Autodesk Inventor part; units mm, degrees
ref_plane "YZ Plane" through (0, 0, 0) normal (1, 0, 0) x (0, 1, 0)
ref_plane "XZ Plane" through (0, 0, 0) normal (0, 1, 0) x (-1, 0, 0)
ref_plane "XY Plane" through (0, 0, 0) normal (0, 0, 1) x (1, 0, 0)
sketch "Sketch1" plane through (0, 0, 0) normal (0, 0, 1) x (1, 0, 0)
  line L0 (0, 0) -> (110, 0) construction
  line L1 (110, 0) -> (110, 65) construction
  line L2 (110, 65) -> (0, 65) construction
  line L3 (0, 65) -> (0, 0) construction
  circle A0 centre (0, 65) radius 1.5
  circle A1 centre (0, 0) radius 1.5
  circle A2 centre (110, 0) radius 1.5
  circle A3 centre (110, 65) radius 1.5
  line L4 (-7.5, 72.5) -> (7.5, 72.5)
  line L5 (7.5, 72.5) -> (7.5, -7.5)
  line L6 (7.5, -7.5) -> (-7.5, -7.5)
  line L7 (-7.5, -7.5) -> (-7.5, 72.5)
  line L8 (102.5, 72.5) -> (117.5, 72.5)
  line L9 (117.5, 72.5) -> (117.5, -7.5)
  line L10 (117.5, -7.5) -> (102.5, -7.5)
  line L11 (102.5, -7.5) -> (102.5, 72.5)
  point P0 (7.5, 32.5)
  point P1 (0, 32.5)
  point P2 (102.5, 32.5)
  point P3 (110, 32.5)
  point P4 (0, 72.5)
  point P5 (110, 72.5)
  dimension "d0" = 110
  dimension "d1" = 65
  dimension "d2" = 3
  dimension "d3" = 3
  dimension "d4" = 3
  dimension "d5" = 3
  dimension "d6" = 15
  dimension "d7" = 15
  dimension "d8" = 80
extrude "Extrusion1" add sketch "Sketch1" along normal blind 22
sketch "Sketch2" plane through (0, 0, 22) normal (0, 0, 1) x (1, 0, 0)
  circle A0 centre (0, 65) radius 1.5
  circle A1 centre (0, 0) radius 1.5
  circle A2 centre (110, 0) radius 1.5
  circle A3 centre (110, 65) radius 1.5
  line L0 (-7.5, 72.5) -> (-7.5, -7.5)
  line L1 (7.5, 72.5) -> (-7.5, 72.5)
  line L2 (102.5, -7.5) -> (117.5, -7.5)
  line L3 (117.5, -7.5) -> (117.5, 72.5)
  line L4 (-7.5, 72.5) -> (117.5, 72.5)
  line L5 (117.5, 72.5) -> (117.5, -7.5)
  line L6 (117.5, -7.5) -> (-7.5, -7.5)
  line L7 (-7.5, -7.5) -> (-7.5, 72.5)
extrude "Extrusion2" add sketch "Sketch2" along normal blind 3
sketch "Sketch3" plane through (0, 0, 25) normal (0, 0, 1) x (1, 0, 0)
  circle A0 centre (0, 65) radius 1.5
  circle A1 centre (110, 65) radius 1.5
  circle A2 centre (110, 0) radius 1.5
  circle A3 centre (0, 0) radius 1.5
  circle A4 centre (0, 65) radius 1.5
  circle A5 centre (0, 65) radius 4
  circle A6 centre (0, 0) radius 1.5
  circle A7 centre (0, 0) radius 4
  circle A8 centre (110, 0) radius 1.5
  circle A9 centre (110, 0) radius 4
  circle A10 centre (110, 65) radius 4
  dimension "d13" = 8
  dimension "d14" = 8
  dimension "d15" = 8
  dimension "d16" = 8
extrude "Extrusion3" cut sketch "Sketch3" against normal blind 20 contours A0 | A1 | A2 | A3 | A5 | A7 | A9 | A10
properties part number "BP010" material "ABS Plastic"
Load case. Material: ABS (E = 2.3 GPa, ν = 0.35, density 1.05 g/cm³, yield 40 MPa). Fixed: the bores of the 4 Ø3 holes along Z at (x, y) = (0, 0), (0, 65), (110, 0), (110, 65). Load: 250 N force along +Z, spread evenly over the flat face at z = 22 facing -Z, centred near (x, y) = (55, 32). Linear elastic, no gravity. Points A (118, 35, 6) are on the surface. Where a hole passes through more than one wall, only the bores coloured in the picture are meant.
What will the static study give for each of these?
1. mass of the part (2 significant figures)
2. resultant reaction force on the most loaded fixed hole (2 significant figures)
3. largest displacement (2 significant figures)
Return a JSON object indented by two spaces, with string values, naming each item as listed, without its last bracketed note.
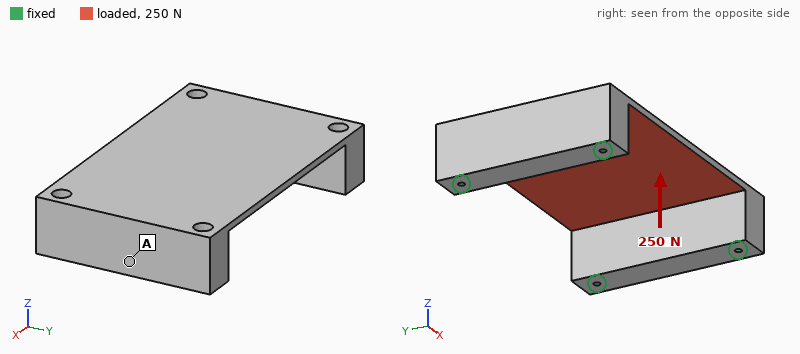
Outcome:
{
  "mass of the part": "83 g",
  "resultant reaction force on the most loaded fixed hole": "94 N",
  "largest displacement": "1.6 mm"
}
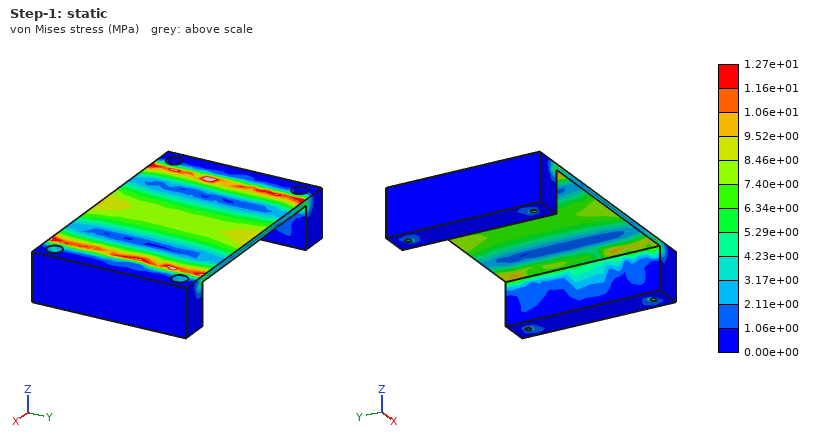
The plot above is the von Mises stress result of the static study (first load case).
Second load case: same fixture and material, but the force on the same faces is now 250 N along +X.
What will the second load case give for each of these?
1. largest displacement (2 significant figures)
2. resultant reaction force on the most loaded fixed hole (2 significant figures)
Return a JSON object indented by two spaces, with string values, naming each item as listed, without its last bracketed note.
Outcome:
{
  "largest displacement": "0.23 mm",
  "resultant reaction force on the most loaded fixed hole": "63 N"
}
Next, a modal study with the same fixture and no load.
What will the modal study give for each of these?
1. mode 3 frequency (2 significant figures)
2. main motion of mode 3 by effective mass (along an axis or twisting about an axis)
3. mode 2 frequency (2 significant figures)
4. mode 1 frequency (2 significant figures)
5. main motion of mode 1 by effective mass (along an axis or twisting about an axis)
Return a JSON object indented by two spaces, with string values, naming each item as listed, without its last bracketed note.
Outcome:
{
  "mode 3 frequency": "790 Hz",
  "main motion of mode 3 by effective mass": "along X",
  "mode 2 frequency": "610 Hz",
  "mode 1 frequency": "490 Hz",
  "main motion of mode 1 by effective mass": "along Z"
}
